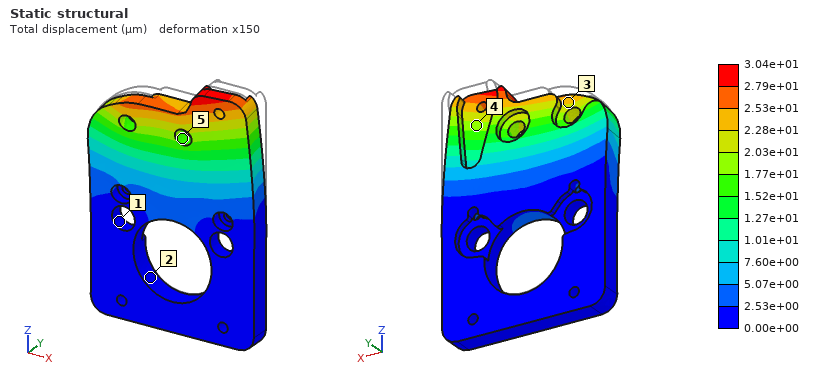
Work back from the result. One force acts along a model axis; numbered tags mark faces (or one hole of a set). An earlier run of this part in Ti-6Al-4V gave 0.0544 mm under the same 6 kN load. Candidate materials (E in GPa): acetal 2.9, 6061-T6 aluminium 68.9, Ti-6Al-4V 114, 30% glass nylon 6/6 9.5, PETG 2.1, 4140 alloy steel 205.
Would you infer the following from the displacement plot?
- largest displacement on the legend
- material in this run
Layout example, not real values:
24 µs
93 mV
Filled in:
3.04e+01 µm
4140 alloy steel
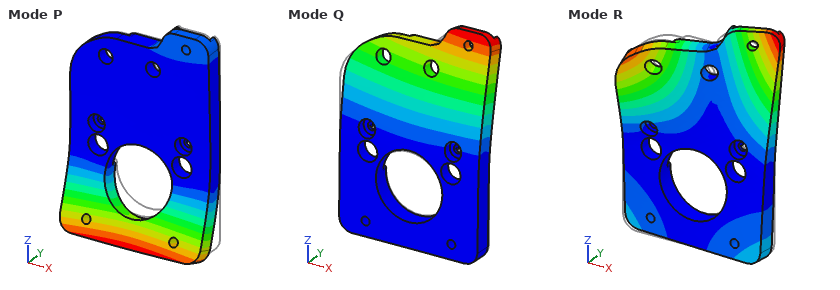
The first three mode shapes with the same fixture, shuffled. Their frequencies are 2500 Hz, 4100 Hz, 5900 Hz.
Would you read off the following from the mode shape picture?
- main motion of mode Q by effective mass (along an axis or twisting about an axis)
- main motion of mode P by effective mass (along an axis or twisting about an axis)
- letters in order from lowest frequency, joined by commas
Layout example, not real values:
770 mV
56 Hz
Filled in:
along Y
along Y
Q, P, R
